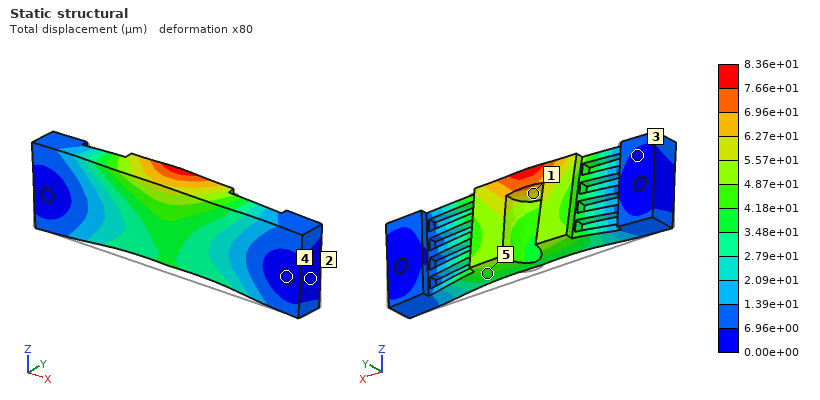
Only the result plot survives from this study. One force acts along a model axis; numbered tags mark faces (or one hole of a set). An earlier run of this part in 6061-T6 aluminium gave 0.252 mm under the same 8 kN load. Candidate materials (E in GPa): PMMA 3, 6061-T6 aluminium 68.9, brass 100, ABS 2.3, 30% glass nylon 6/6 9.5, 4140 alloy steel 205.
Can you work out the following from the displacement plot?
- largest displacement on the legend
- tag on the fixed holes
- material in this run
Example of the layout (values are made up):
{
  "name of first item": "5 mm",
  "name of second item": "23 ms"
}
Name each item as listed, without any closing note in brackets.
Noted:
{
  "largest displacement on the legend": "8.36e+01 µm",
  "tag on the fixed holes": "4",
  "material in this run": "4140 alloy steel"
}
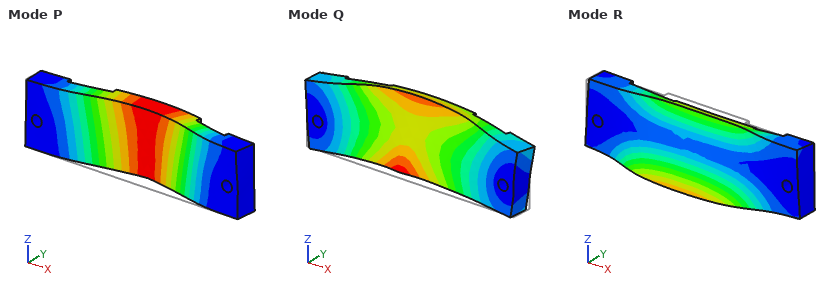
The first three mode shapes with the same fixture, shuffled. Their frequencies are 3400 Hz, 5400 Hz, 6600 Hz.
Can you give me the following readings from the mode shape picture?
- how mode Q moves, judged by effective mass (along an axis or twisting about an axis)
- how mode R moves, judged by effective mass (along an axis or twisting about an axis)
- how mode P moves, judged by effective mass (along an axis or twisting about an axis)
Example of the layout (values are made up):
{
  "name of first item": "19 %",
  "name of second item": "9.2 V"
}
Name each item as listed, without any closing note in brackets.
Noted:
{
  "how mode Q moves, judged by effective mass": "along Z",
  "how mode R moves, judged by effective mass": "along Z",
  "how mode P moves, judged by effective mass": "along Y"
}
